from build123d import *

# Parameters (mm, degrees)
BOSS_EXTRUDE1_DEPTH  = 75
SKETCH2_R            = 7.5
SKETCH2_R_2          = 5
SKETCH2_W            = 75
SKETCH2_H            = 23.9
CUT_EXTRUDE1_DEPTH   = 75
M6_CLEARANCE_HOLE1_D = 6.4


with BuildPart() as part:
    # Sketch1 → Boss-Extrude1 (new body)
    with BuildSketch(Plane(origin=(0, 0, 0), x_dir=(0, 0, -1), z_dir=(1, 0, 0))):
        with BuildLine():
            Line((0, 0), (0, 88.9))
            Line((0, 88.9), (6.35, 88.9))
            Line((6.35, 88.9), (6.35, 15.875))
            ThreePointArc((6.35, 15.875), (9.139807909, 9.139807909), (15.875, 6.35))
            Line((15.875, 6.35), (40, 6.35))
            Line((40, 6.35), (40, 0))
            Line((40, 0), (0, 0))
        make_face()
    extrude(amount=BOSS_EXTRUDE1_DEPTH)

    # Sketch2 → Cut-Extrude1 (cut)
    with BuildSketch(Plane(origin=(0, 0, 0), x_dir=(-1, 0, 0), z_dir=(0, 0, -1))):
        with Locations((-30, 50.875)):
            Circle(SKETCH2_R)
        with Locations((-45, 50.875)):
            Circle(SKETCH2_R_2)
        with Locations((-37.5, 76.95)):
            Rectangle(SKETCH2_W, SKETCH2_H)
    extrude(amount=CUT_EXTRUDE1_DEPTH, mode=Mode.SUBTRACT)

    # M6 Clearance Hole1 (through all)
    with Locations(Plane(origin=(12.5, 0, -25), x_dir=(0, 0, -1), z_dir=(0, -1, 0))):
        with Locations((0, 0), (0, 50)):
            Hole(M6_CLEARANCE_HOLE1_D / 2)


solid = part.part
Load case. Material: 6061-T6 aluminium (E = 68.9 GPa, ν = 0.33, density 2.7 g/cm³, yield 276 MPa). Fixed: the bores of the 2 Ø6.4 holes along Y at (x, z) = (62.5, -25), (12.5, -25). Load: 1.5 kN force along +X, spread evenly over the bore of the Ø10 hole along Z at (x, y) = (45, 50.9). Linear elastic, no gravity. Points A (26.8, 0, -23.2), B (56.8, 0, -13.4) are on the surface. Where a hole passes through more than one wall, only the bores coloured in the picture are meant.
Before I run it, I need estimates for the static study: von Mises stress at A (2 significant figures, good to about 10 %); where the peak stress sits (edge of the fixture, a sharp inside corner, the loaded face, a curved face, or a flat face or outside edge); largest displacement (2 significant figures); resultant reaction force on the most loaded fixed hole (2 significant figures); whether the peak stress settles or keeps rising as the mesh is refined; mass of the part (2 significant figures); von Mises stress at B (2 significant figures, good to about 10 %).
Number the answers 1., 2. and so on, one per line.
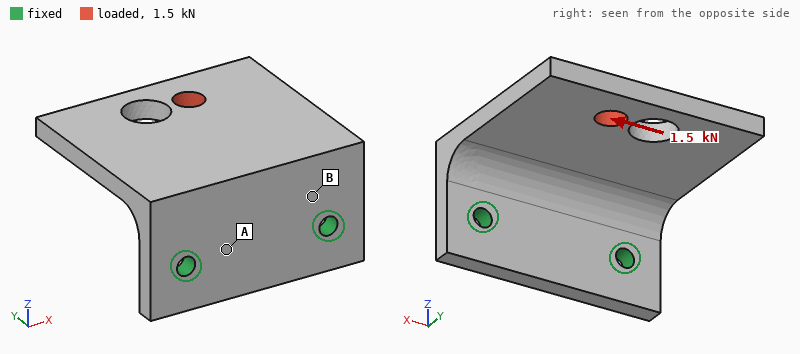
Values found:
1. 11 MPa
2. edge of the fixture
3. 0.15 mm
4. 1.6 kN
5. keeps rising
6. 130 g
7. 25 MPa
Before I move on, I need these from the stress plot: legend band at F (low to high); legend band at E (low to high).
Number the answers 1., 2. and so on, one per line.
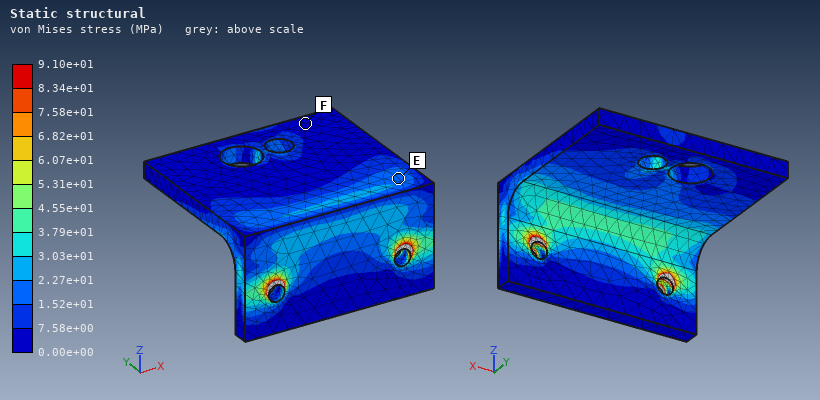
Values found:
1. 0.00e+00 to 7.58e+00 MPa
2. 1.52e+01 to 2.27e+01 MPa
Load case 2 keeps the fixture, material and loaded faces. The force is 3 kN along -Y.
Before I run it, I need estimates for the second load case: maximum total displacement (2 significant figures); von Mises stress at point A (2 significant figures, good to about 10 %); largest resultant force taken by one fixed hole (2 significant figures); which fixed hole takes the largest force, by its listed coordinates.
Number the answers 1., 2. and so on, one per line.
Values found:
1. 0.45 mm
2. 43 MPa
3. 1.9 kN
4. (62.5, -25)
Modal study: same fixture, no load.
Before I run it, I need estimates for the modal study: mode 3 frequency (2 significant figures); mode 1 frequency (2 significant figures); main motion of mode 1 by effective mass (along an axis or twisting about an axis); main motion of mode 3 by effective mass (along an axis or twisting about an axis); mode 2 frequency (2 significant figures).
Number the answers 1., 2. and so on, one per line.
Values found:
1. 3500 Hz
2. 1100 Hz
3. along Z
4. along X
5. 2300 Hz
